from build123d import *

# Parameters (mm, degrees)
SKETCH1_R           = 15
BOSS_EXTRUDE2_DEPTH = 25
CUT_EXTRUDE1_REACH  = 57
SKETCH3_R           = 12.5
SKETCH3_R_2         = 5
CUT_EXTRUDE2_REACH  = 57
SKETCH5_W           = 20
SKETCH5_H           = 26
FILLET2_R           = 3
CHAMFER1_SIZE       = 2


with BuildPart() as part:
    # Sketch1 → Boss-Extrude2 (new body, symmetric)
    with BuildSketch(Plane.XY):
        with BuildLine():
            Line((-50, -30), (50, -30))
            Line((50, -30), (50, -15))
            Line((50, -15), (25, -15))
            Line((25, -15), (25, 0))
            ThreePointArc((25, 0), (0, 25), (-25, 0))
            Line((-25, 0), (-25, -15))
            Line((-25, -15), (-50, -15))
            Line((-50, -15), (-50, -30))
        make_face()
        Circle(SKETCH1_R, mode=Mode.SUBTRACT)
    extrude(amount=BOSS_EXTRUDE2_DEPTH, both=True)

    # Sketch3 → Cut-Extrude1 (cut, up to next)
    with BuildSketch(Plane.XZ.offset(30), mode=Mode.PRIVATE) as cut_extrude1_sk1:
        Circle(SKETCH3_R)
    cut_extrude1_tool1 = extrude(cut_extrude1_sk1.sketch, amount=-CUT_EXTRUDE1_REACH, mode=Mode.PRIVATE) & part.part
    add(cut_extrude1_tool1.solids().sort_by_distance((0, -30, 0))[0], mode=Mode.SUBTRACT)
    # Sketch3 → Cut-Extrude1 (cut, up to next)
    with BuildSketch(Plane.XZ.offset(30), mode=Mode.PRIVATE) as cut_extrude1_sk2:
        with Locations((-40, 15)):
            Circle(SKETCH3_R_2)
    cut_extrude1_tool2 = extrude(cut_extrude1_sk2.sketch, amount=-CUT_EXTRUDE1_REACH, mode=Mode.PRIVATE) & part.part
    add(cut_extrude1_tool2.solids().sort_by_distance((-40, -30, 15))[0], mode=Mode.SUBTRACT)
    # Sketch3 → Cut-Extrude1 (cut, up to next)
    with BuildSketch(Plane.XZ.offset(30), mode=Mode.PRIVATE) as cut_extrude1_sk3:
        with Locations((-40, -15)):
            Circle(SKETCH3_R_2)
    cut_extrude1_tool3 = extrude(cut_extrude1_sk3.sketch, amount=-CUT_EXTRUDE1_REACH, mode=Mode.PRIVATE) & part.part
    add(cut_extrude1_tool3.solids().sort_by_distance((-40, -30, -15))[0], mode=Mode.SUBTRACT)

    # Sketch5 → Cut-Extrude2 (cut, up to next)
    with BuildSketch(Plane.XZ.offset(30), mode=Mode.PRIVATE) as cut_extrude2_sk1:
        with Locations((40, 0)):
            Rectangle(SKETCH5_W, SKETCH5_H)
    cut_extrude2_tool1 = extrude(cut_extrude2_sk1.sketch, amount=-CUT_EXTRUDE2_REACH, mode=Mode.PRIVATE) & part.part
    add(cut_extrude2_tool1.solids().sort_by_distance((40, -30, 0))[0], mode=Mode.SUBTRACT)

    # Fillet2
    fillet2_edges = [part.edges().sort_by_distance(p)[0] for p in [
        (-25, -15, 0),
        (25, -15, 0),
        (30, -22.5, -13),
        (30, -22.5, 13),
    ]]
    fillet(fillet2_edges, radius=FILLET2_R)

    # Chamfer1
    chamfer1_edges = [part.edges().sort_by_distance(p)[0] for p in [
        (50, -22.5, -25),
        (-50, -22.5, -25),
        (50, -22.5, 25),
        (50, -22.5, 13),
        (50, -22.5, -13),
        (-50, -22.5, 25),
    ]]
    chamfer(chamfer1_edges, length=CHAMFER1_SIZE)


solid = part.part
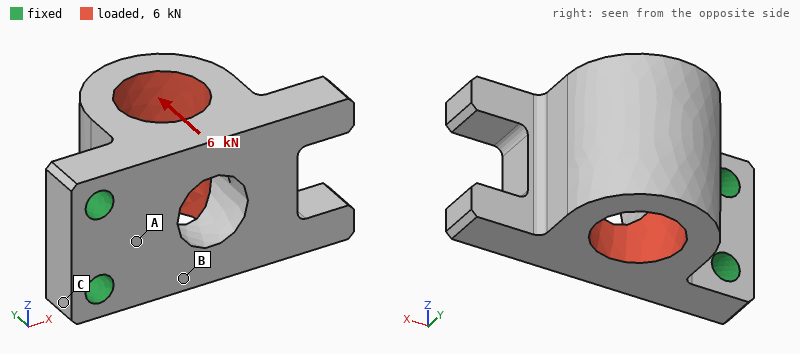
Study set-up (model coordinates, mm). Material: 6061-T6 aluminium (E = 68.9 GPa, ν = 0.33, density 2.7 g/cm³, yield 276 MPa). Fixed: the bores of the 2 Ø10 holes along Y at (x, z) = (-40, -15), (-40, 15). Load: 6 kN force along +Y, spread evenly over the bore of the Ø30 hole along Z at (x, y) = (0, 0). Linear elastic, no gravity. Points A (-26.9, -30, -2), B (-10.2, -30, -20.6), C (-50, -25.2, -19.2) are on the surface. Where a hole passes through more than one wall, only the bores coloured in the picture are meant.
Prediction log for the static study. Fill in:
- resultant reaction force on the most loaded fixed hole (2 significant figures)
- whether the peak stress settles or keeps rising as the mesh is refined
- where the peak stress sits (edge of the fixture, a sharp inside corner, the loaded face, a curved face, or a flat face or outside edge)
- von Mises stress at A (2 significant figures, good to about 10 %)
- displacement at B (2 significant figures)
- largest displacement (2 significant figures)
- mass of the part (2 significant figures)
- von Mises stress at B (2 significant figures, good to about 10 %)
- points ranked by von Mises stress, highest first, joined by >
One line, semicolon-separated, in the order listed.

3.0 kN; keeps rising; edge of the fixture; 57 MPa; 0.079 mm; 0.34 mm; 290 g; 34 MPa; A > B > C
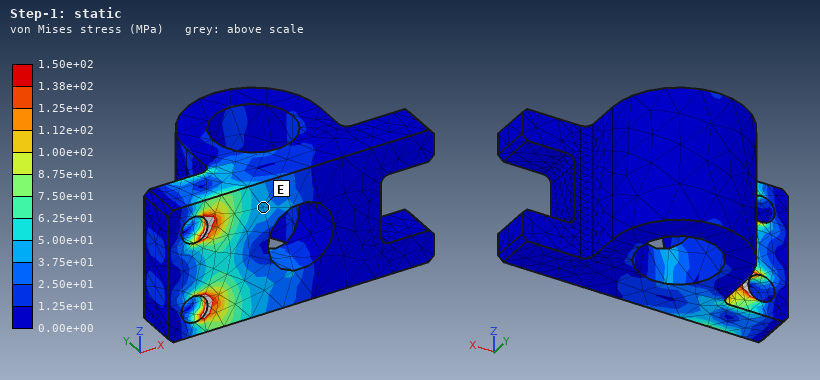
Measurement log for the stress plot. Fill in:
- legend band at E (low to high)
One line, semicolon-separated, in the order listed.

3.75e+01 to 5.00e+01 MPa
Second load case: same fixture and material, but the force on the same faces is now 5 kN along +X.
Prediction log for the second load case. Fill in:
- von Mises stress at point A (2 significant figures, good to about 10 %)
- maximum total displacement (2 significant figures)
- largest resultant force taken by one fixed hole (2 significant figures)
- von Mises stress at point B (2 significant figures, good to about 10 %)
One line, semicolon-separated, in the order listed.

40 MPa; 0.23 mm; 2.5 kN; 19 MPa
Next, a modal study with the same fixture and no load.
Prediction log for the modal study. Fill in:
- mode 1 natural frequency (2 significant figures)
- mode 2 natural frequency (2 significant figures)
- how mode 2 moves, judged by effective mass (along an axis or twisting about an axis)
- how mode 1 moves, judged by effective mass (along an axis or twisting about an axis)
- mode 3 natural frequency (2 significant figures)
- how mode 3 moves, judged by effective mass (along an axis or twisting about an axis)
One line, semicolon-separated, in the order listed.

1500 Hz; 3400 Hz; along Z; along Y; 4400 Hz; twisting about X
